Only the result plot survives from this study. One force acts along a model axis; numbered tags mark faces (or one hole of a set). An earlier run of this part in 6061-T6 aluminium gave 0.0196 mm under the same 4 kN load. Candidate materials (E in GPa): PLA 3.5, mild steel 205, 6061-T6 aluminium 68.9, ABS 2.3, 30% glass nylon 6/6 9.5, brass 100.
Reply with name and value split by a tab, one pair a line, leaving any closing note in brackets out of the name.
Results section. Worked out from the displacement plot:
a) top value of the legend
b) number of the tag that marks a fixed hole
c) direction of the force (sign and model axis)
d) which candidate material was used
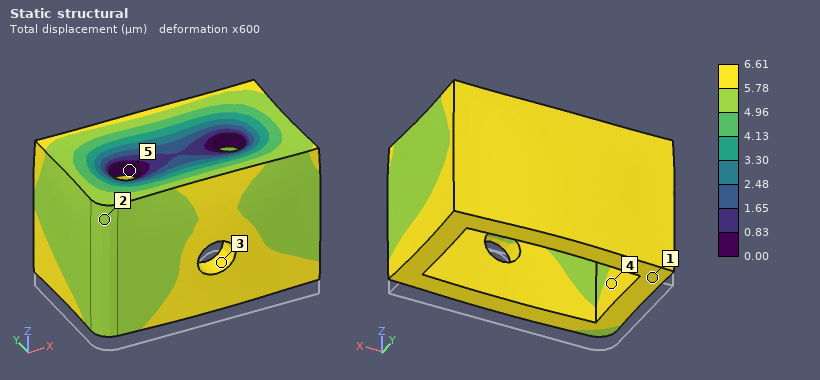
top value of the legend	6.61 µm
number of the tag that marks a fixed hole	5
direction of the force	+Z
which candidate material was used	mild steel
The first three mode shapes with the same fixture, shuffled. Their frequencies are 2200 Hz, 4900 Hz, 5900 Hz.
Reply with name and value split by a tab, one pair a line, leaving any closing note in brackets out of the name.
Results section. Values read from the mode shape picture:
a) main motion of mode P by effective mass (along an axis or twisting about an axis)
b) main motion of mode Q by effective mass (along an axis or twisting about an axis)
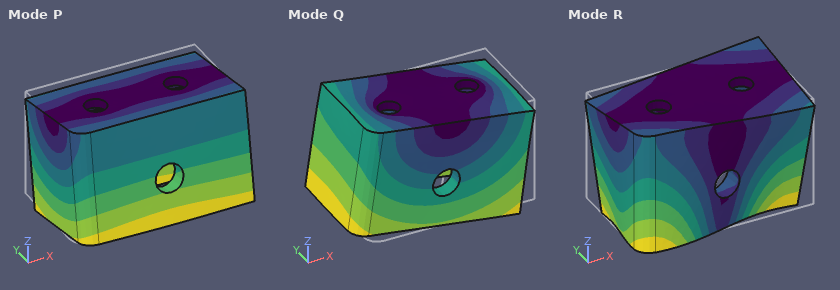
main motion of mode P by effective mass	along Y
main motion of mode Q by effective mass	along X
